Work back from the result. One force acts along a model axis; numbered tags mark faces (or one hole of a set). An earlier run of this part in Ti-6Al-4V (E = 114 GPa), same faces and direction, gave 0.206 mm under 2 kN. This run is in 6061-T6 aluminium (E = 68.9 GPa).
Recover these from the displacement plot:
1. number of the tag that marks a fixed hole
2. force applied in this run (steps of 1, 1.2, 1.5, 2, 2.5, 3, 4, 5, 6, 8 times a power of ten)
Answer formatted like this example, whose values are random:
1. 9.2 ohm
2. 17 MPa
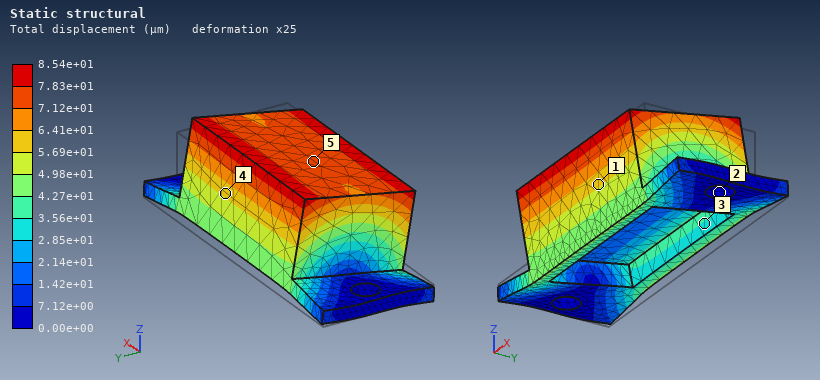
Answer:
1. 2
2. 500 N
